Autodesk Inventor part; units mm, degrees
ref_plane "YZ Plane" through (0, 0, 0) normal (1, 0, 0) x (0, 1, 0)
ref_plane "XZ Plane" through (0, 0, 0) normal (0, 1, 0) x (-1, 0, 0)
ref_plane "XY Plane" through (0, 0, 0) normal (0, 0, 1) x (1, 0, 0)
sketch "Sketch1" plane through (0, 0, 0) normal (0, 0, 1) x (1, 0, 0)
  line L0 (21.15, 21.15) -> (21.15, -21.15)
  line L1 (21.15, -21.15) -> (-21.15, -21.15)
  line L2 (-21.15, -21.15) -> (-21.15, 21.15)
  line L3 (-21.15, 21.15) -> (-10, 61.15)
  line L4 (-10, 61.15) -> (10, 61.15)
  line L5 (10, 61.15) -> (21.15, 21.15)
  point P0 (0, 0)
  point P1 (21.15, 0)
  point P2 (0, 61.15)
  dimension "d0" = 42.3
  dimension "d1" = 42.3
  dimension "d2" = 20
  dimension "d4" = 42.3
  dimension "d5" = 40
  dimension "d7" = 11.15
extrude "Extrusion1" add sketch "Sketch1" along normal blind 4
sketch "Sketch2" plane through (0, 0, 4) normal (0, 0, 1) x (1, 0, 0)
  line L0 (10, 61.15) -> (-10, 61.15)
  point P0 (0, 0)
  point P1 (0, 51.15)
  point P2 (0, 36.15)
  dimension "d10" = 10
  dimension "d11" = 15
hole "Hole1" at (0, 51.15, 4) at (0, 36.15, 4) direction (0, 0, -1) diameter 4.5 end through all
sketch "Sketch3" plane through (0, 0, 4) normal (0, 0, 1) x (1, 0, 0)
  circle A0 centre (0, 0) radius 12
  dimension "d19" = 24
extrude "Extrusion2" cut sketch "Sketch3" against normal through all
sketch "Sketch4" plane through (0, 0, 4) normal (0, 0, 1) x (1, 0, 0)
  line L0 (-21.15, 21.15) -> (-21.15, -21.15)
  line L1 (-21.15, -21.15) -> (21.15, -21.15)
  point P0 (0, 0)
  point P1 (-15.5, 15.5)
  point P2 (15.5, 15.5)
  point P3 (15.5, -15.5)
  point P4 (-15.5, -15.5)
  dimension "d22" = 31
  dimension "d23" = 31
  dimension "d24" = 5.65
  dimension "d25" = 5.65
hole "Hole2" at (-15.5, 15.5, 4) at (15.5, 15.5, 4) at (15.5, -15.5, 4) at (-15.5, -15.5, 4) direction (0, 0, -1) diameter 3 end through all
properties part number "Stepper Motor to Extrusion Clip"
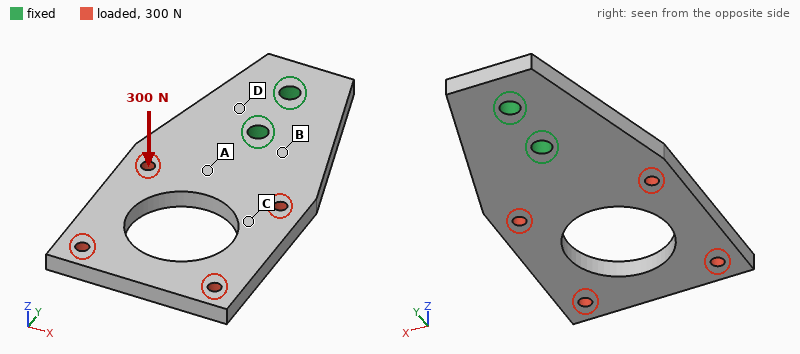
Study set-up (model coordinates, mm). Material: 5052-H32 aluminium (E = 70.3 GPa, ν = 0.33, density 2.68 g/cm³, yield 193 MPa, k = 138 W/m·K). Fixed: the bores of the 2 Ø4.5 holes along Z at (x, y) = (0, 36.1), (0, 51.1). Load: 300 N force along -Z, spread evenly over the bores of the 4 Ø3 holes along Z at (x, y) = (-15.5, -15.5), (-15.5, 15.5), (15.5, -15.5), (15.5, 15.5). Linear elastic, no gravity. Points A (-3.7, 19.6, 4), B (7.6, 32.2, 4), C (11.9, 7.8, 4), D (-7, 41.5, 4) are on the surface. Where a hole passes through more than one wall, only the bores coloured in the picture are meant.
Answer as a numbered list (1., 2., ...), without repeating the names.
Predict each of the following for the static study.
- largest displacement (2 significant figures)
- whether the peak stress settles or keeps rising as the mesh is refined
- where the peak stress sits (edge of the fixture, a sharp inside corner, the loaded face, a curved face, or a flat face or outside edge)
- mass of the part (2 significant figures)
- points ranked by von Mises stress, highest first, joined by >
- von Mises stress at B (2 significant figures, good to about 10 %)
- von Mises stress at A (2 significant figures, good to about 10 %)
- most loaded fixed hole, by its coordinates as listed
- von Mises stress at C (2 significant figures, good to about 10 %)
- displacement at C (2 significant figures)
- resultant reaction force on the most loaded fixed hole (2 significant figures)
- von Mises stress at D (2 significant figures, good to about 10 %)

1. 0.82 mm
2. keeps rising
3. edge of the fixture
4. 27 g
5. B > C > A > D
6. 82 MPa
7. 45 MPa
8. (0, 36.1)
9. 64 MPa
10. 0.26 mm
11. 590 N
12. 26 MPa
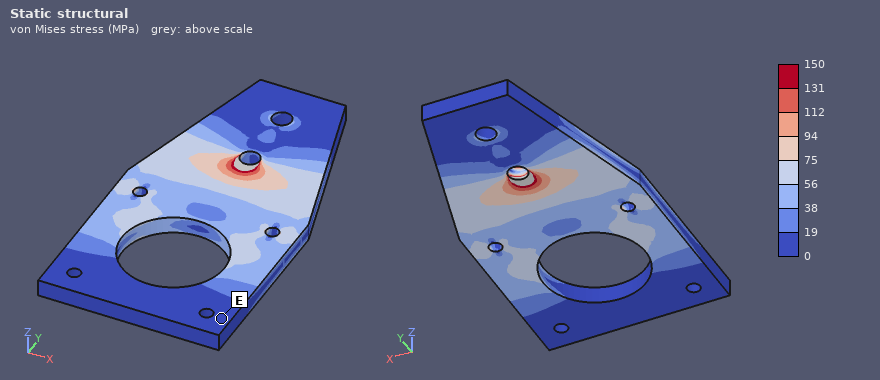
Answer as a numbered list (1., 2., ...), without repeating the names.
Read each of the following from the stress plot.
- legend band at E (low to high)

1. 0 to 19 MPa
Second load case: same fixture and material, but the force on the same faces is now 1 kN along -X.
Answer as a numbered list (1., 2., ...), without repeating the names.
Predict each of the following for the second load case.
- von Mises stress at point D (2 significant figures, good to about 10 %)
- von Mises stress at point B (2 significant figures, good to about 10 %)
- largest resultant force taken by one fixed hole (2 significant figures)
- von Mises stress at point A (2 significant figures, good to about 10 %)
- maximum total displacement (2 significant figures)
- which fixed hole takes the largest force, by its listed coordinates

1. 33 MPa
2. 26 MPa
3. 2.8 kN
4. 22 MPa
5. 0.12 mm
6. (0, 36.1)
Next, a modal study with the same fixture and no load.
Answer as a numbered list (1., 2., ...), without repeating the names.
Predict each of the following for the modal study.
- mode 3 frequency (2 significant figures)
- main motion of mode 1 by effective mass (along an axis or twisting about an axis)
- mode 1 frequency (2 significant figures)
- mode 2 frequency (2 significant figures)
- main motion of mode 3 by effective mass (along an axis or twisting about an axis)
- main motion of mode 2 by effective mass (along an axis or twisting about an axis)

1. 4400 Hz
2. along Z
3. 990 Hz
4. 2200 Hz
5. along X
6. twisting about Y
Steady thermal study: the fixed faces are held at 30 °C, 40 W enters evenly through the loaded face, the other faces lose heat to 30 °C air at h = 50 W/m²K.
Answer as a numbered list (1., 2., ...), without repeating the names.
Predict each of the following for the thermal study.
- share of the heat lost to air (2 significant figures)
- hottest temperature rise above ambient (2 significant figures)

1. 27 %
2. 78 K
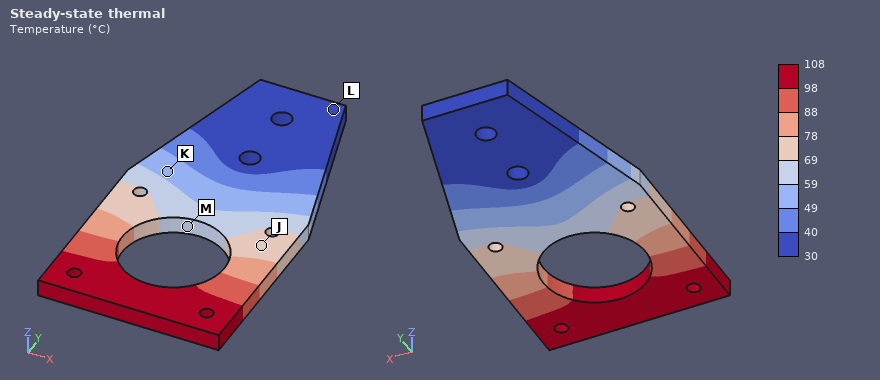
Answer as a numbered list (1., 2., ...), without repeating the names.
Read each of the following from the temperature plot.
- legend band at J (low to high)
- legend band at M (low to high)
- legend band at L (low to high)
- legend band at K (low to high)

1. 69 to 78 °C
2. 59 to 69 °C
3. 30 to 40 °C
4. 49 to 59 °C
